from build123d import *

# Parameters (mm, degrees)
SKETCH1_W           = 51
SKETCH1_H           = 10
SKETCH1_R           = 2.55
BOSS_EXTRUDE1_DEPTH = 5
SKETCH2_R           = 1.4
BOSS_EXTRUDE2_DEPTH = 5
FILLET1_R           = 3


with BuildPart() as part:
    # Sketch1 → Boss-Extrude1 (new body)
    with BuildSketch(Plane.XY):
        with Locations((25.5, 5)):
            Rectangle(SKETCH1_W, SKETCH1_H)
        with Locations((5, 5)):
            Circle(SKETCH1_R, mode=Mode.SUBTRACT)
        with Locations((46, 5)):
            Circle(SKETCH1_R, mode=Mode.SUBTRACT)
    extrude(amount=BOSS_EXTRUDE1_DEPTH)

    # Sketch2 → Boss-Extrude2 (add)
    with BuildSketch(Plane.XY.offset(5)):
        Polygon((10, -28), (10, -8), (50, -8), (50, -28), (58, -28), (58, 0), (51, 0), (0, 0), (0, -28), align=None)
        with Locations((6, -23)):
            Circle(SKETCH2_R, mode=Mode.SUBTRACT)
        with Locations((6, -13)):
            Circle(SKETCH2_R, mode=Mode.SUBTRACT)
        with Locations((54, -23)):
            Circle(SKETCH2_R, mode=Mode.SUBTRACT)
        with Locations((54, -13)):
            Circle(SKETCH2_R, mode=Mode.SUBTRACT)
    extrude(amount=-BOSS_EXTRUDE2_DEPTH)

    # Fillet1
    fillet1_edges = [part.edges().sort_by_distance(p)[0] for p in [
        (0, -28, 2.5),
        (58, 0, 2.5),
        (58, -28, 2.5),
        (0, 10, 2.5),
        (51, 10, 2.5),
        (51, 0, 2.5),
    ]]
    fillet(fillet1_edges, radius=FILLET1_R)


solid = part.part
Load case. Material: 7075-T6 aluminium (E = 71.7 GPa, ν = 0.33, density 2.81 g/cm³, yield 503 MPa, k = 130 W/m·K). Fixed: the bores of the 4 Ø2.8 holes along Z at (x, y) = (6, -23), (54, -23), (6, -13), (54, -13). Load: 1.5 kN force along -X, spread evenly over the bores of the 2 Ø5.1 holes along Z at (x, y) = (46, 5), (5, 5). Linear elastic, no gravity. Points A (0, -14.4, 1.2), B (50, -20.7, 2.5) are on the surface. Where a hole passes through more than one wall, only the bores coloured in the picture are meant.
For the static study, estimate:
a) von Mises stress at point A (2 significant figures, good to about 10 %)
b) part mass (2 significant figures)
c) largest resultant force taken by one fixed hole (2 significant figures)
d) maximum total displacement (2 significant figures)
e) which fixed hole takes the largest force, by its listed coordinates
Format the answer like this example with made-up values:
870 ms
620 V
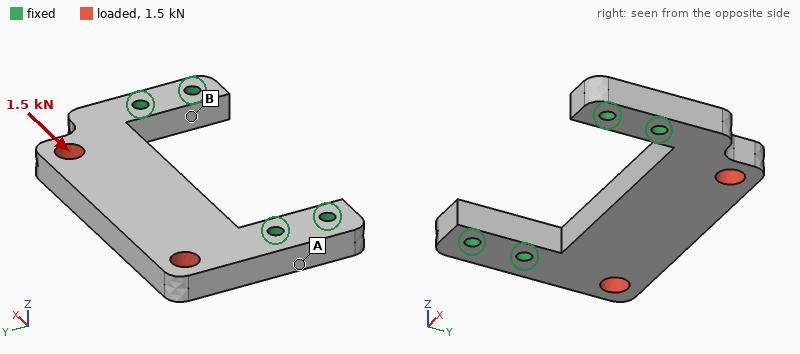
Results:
34 MPa
18 g
1.0 kN
18 µm
(6, -13)
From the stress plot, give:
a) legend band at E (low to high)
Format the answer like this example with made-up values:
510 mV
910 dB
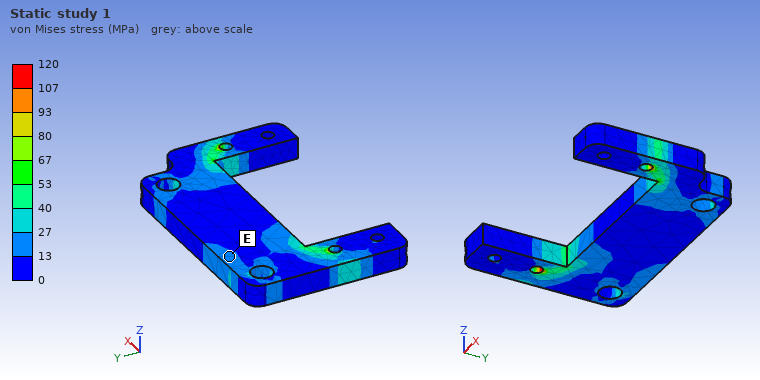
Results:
13 to 27 MPa
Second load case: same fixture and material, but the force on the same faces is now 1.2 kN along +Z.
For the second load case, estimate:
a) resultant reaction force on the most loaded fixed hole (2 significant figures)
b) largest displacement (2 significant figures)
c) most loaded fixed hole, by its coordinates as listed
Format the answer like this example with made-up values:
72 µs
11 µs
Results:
940 N
0.26 mm
(6, -13)
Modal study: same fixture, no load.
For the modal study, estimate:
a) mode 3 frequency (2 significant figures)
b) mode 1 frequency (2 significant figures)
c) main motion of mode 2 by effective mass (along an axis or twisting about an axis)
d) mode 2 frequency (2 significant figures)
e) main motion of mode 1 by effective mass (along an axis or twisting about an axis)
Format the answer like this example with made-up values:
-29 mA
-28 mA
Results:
12 kHz
4100 Hz
twisting about Y
9500 Hz
along Z
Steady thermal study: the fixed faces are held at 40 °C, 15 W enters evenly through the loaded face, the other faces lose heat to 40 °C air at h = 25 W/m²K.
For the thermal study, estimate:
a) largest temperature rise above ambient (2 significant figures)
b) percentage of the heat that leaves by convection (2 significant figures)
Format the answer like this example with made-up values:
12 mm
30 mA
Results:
21 K
6.2 %
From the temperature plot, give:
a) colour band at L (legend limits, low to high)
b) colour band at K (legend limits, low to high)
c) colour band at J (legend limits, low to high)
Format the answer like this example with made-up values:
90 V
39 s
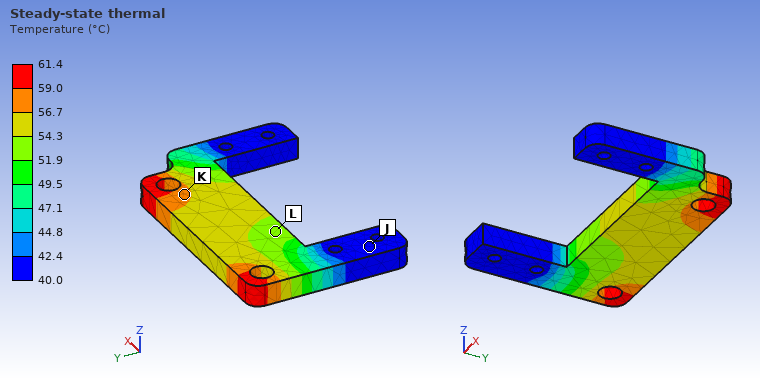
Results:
51.9 to 54.3 °C
56.7 to 59.0 °C
40.0 to 42.4 °C
